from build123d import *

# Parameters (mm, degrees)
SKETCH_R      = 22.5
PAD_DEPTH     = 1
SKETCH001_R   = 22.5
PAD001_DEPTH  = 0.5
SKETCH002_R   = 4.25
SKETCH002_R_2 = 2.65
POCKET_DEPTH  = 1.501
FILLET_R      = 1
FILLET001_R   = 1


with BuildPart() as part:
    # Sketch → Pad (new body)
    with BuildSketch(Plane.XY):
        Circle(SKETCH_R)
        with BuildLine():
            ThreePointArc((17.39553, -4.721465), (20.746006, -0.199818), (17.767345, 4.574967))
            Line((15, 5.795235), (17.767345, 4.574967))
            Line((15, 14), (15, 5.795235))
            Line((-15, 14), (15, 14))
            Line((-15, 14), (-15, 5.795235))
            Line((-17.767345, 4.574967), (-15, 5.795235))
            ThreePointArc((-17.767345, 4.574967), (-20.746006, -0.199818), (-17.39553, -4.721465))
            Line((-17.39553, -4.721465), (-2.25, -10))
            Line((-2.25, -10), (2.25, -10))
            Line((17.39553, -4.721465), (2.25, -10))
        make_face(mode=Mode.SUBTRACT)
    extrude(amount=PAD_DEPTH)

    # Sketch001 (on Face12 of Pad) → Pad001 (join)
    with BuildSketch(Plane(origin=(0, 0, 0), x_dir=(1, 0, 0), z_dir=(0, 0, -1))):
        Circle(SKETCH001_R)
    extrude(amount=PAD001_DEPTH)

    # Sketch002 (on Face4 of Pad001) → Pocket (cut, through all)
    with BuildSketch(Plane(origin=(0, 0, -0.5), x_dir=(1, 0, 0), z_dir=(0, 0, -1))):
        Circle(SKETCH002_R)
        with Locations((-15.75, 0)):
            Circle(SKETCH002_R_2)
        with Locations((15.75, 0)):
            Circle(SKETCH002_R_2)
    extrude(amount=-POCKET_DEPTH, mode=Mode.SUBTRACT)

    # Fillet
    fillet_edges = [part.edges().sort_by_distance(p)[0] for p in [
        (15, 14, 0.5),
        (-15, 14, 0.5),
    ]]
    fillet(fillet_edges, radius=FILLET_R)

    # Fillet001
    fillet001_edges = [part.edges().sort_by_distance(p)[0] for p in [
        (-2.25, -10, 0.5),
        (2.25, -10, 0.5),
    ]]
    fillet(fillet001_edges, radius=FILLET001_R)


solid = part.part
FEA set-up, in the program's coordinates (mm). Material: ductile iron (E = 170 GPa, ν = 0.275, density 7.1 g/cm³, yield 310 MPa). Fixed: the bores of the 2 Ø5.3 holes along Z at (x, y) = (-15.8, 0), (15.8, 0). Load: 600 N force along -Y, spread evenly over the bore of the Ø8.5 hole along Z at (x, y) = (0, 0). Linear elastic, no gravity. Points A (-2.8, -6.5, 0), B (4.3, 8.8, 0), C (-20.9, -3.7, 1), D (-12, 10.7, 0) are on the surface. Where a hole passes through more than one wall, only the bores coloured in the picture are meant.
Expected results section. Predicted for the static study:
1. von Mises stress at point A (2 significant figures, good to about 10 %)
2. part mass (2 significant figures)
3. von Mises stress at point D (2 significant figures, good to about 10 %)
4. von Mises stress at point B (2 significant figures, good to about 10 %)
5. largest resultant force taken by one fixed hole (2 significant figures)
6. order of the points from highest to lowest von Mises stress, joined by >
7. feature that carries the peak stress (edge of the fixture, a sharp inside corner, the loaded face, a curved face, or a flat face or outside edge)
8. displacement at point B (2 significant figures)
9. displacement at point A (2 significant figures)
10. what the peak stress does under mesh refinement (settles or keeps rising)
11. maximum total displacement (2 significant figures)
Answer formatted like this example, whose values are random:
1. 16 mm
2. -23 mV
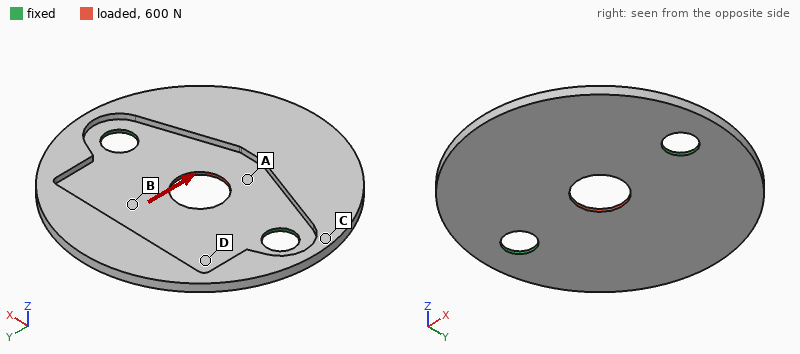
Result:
1. 45 MPa
2. 11 g
3. 23 MPa
4. 36 MPa
5. 300 N
6. A > B > D > C
7. edge of the fixture
8. 4.7 µm
9. 8.5 µm
10. keeps rising
11. 10 µm
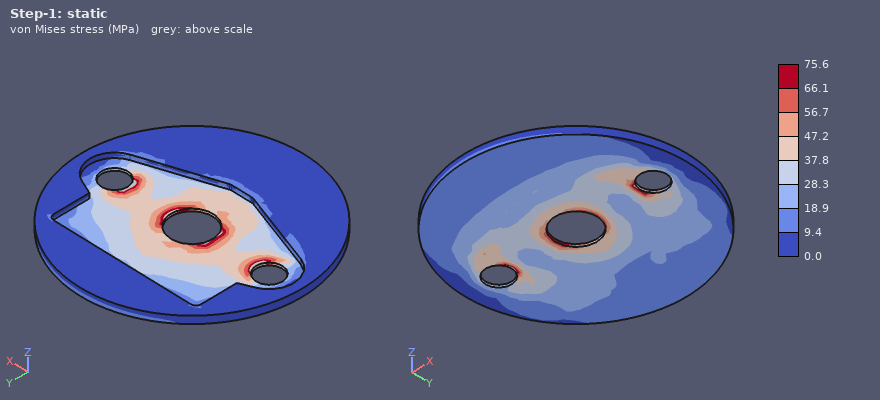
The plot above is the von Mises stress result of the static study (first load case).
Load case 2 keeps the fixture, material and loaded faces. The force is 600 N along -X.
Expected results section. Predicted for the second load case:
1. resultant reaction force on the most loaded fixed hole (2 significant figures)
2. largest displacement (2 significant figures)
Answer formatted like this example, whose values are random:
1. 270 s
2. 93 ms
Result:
1. 300 N
2. 3.7 µm
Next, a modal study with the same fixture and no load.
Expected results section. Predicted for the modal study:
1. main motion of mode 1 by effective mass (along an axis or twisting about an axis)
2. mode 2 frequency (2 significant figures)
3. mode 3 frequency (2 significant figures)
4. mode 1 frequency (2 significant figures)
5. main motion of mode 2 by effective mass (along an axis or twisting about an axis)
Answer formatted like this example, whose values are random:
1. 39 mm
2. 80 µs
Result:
1. twisting about X
2. 1500 Hz
3. 3700 Hz
4. 1200 Hz
5. along Z
